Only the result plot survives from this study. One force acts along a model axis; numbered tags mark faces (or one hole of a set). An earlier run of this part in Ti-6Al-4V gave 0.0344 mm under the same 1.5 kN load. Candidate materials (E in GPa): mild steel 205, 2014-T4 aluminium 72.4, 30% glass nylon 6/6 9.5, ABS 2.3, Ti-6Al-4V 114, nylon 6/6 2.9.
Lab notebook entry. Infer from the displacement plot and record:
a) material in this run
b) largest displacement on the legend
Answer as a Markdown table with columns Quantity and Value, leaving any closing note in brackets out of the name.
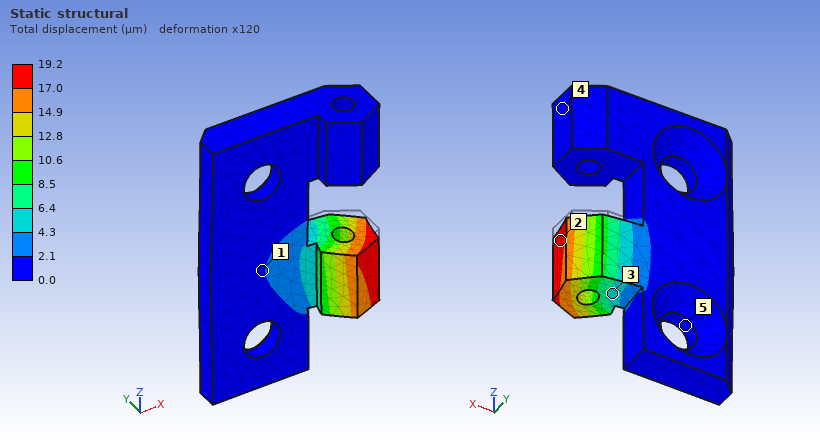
| Quantity | Value |
|---|---|
| material in this run | mild steel |
| largest displacement on the legend | 19.2 µm |
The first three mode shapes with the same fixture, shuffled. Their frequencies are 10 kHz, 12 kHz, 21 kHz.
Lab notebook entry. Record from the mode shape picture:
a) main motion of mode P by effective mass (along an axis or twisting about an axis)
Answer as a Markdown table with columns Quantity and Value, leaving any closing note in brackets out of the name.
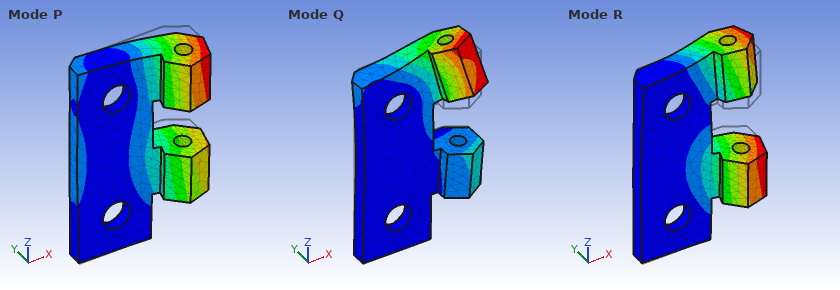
| Quantity | Value |
|---|---|
| main motion of mode P by effective mass | along Y |
